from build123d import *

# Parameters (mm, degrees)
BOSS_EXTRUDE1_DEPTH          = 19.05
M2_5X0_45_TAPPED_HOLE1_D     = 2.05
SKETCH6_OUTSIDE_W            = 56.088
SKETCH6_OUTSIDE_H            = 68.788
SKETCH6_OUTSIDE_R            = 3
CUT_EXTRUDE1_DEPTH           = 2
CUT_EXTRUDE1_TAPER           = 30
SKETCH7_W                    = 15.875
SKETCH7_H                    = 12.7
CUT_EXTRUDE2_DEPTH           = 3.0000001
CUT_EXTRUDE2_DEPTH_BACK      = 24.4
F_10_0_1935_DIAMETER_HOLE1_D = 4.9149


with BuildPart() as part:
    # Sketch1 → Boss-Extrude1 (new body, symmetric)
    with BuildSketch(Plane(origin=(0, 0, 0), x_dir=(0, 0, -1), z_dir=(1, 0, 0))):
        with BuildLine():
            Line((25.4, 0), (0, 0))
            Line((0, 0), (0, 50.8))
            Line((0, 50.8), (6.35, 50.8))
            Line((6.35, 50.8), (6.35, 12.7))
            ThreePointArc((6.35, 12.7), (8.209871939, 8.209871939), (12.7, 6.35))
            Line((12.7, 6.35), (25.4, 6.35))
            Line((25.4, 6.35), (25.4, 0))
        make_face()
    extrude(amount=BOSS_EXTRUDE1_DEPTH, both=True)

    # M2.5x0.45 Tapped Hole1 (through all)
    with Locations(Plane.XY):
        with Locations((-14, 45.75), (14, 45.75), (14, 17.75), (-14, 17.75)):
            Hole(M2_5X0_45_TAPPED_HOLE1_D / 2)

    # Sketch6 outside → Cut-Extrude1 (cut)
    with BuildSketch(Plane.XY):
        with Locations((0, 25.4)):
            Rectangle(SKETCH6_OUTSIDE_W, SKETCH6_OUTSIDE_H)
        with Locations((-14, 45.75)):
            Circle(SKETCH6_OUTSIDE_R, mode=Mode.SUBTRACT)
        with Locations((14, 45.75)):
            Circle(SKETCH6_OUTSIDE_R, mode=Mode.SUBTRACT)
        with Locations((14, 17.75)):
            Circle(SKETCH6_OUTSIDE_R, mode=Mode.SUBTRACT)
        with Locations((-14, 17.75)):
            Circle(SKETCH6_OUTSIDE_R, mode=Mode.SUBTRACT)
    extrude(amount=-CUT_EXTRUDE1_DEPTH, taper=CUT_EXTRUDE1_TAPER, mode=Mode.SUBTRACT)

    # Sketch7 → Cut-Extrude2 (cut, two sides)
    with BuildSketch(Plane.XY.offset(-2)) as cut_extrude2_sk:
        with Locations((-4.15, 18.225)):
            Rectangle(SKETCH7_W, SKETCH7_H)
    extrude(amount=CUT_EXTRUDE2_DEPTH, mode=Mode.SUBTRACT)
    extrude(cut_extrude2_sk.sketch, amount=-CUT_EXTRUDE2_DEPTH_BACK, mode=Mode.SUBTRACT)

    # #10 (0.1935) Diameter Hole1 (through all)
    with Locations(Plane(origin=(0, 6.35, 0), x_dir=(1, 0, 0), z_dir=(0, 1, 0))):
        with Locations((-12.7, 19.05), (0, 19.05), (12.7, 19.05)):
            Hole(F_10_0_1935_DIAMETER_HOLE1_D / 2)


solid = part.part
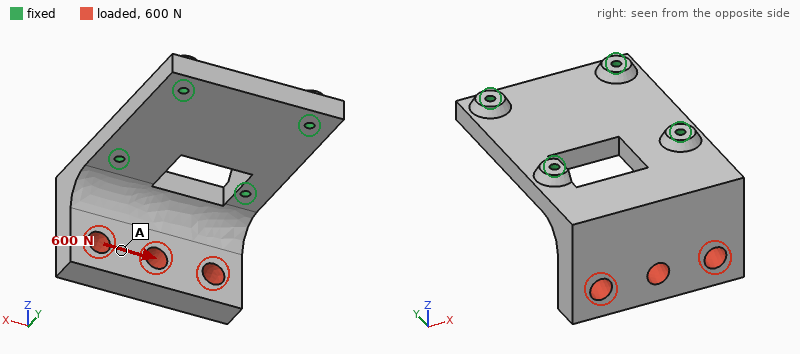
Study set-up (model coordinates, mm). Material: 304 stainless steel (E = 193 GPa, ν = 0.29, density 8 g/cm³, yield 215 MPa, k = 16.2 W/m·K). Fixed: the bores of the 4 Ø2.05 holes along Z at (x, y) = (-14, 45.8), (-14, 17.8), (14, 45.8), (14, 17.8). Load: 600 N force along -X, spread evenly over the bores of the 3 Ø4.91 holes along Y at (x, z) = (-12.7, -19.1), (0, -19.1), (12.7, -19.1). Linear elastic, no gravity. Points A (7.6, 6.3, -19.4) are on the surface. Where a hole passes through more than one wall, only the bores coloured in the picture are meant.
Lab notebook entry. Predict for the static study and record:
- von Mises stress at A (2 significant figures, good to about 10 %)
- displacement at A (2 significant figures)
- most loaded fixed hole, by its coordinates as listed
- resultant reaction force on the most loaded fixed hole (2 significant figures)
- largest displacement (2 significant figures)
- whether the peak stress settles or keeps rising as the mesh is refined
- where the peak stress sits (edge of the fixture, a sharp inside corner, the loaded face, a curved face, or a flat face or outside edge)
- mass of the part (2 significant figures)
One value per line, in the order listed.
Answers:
9.7 MPa
6.5 µm
(14, 17.8)
590 N
10 µm
keeps rising
edge of the fixture
99 g
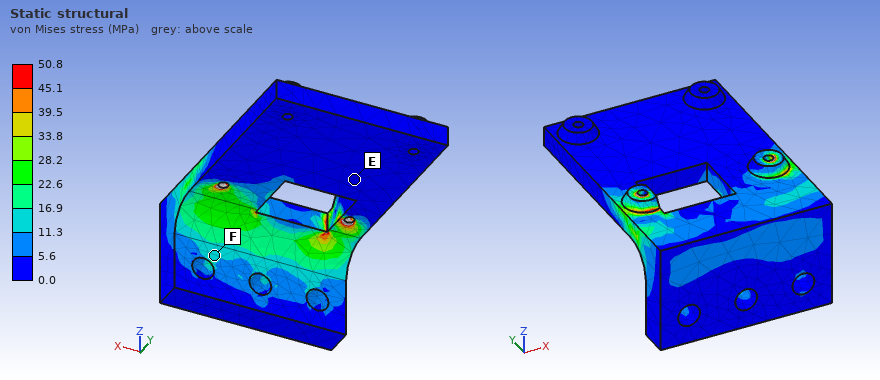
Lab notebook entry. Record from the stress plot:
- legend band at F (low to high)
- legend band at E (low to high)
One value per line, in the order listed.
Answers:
11.3 to 16.9 MPa
0.0 to 5.6 MPa
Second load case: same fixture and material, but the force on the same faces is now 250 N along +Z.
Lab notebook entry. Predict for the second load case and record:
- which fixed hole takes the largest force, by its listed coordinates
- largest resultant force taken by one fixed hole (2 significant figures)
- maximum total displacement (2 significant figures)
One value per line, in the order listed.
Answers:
(14, 17.8)
150 N
18 µm
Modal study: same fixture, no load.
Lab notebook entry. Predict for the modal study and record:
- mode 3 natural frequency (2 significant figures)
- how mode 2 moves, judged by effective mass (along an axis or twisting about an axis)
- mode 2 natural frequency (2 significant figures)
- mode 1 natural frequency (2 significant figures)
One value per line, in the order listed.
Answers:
12 kHz
along X
7600 Hz
2900 Hz
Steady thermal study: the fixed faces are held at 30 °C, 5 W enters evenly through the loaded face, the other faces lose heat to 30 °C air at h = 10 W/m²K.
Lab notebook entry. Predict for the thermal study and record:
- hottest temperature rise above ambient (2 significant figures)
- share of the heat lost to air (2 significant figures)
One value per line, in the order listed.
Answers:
47 K
21 %
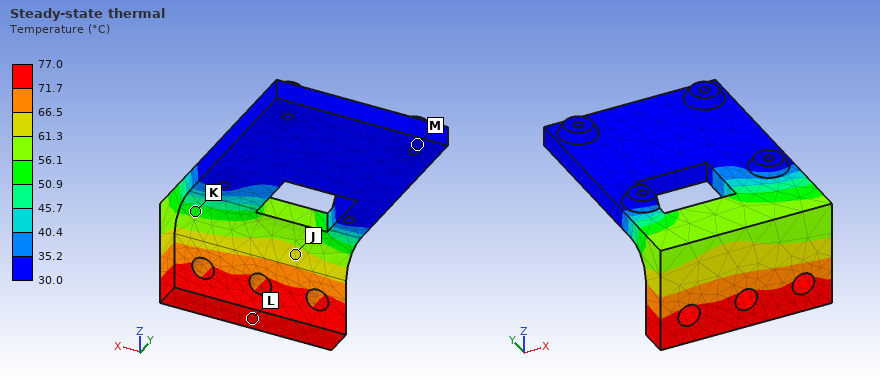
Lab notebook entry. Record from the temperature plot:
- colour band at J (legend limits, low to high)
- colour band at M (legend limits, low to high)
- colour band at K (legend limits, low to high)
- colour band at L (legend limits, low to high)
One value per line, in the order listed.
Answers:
61.3 to 66.5 °C
30.0 to 35.2 °C
50.9 to 56.1 °C
71.7 to 77.0 °C
